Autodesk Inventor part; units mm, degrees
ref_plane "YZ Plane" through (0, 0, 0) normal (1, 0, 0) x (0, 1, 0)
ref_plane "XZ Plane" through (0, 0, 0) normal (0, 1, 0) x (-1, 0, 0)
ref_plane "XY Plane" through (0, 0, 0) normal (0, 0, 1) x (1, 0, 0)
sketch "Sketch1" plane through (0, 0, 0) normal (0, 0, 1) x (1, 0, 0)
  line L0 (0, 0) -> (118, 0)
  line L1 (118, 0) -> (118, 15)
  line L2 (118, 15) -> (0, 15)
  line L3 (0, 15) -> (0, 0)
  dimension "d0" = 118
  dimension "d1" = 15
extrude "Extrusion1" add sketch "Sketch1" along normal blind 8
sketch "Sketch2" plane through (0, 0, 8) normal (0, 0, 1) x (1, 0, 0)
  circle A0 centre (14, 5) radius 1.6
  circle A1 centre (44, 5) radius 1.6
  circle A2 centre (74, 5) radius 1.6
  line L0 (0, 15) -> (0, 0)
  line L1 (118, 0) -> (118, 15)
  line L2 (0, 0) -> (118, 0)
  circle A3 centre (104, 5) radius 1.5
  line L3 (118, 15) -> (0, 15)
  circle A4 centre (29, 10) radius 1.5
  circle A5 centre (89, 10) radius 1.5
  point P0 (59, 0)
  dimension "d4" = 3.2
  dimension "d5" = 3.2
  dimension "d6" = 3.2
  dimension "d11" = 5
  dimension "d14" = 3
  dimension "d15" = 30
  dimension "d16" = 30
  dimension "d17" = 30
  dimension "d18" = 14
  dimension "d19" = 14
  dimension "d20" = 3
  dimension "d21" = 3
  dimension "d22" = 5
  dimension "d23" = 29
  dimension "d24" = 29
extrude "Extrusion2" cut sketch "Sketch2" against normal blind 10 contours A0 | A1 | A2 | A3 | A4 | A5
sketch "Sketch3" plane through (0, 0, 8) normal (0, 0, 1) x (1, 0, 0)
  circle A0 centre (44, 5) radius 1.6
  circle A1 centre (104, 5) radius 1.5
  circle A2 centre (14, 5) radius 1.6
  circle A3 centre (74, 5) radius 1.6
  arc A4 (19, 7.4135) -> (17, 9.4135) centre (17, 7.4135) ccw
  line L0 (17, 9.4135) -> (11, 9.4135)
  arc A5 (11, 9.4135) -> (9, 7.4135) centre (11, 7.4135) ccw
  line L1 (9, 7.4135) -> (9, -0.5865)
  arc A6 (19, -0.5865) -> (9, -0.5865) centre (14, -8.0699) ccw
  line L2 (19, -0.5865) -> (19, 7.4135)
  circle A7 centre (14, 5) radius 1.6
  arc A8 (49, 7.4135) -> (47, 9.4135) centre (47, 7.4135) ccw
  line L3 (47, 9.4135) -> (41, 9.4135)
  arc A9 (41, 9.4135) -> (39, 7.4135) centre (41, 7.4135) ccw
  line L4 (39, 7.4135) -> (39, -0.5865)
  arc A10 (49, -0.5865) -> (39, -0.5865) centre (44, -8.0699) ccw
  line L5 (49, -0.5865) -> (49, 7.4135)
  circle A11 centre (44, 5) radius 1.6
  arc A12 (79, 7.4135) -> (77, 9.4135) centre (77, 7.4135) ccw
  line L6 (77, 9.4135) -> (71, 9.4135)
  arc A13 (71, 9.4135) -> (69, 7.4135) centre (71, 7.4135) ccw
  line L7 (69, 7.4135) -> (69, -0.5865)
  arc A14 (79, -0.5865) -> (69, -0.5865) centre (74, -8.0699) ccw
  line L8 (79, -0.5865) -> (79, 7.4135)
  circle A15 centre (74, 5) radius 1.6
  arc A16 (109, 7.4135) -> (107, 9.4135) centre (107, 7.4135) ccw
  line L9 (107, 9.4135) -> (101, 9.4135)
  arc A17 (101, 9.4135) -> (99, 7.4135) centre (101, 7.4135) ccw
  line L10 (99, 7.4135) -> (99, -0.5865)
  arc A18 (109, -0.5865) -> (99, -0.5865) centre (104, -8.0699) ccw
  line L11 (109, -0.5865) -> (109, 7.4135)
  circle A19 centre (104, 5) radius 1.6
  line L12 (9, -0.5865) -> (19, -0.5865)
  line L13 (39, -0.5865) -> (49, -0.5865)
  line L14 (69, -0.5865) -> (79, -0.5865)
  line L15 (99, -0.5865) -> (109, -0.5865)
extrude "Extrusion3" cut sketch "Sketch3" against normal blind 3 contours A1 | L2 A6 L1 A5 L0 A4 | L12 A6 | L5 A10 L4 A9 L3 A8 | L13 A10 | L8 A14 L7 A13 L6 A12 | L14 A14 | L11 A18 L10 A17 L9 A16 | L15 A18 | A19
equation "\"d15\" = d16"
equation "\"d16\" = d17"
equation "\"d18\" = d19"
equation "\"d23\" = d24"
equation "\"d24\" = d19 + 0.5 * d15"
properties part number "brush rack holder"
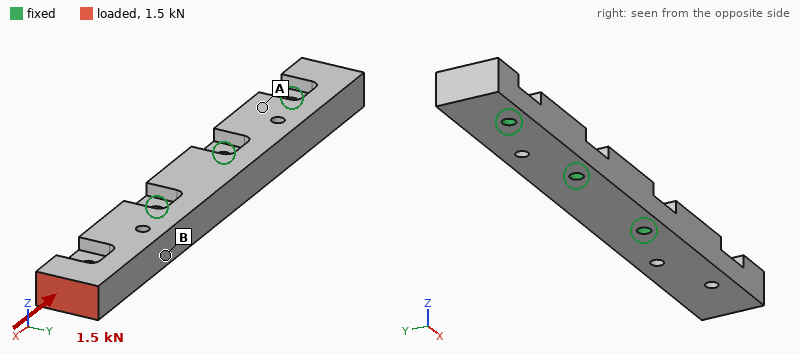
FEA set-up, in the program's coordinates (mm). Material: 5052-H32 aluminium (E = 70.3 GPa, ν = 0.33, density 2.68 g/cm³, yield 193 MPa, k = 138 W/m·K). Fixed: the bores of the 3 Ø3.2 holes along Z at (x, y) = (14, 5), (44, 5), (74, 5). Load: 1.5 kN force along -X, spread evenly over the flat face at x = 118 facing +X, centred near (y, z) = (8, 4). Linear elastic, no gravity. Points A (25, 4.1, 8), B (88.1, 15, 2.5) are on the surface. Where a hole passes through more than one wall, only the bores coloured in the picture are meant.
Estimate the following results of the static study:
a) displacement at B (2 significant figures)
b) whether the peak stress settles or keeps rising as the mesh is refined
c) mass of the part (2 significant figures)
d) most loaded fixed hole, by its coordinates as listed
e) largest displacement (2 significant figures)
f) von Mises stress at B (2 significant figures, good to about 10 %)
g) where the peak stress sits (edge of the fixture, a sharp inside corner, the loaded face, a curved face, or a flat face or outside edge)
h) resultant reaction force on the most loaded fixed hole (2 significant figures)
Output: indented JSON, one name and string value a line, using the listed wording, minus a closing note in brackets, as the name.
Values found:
{
  "displacement at B": "8.4 µm",
  "whether the peak stress settles or keeps rising as the mesh is refined": "keeps rising",
  "mass of the part": "34 g",
  "most loaded fixed hole, by its coordinates as listed": "(74, 5)",
  "largest displacement": "43 µm",
  "von Mises stress at B": "13 MPa",
  "where the peak stress sits": "edge of the fixture",
  "resultant reaction force on the most loaded fixed hole": "1.2 kN"
}
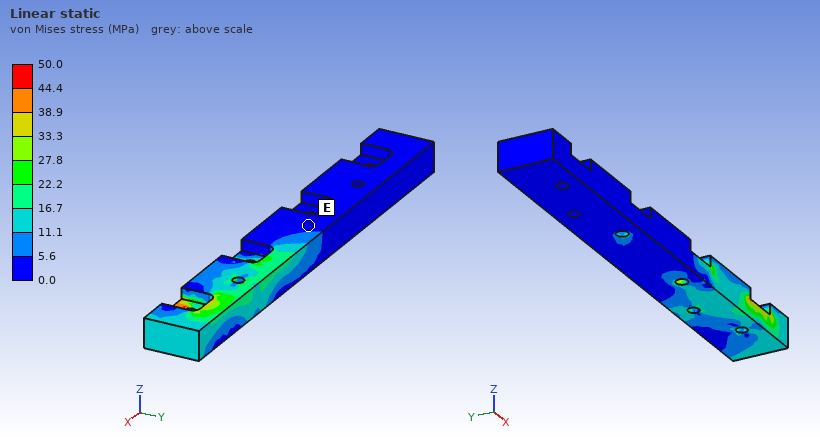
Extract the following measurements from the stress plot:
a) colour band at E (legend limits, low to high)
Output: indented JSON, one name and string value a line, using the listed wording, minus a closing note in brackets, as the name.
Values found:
{
  "colour band at E": "0.0 to 5.6 MPa"
}
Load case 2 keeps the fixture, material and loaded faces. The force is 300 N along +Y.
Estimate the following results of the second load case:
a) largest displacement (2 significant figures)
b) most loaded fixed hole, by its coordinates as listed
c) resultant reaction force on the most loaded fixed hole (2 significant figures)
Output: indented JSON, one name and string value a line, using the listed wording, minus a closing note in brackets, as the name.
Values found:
{
  "largest displacement": "0.12 mm",
  "most loaded fixed hole, by its coordinates as listed": "(74, 5)",
  "resultant reaction force on the most loaded fixed hole": "780 N"
}
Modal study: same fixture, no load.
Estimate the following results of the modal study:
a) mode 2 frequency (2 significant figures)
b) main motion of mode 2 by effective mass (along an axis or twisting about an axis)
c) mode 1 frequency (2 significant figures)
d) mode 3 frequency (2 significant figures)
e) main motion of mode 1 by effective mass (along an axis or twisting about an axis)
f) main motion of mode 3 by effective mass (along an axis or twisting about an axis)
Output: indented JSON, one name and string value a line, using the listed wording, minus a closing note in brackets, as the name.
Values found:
{
  "mode 2 frequency": "4500 Hz",
  "main motion of mode 2 by effective mass": "along Y",
  "mode 1 frequency": "2500 Hz",
  "mode 3 frequency": "11 kHz",
  "main motion of mode 1 by effective mass": "along Z",
  "main motion of mode 3 by effective mass": "twisting about X"
}
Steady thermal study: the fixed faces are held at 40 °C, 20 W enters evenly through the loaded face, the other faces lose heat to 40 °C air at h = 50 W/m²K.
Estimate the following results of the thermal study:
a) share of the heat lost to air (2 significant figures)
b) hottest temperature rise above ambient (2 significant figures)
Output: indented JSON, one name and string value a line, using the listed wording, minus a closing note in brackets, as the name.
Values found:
{
  "share of the heat lost to air": "17 %",
  "hottest temperature rise above ambient": "59 K"
}
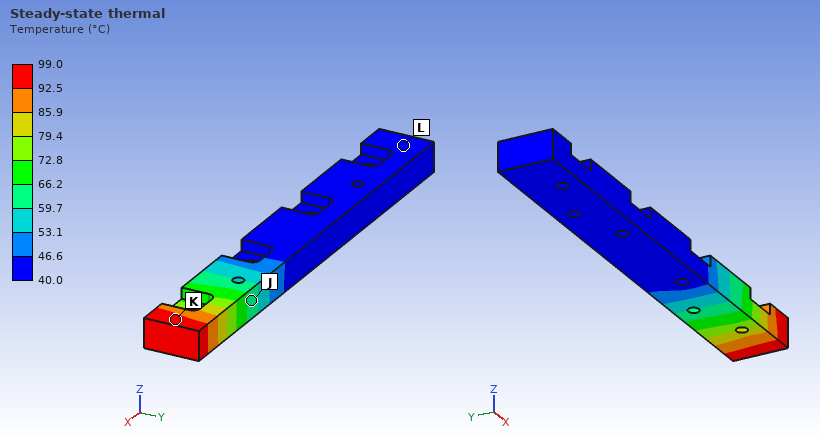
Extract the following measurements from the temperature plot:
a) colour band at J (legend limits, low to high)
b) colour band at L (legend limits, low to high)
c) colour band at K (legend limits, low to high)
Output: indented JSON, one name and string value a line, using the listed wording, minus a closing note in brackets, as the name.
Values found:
{
  "colour band at J": "59.7 to 66.2 °C",
  "colour band at L": "40.0 to 46.6 °C",
  "colour band at K": "92.5 to 99.0 °C"
}
